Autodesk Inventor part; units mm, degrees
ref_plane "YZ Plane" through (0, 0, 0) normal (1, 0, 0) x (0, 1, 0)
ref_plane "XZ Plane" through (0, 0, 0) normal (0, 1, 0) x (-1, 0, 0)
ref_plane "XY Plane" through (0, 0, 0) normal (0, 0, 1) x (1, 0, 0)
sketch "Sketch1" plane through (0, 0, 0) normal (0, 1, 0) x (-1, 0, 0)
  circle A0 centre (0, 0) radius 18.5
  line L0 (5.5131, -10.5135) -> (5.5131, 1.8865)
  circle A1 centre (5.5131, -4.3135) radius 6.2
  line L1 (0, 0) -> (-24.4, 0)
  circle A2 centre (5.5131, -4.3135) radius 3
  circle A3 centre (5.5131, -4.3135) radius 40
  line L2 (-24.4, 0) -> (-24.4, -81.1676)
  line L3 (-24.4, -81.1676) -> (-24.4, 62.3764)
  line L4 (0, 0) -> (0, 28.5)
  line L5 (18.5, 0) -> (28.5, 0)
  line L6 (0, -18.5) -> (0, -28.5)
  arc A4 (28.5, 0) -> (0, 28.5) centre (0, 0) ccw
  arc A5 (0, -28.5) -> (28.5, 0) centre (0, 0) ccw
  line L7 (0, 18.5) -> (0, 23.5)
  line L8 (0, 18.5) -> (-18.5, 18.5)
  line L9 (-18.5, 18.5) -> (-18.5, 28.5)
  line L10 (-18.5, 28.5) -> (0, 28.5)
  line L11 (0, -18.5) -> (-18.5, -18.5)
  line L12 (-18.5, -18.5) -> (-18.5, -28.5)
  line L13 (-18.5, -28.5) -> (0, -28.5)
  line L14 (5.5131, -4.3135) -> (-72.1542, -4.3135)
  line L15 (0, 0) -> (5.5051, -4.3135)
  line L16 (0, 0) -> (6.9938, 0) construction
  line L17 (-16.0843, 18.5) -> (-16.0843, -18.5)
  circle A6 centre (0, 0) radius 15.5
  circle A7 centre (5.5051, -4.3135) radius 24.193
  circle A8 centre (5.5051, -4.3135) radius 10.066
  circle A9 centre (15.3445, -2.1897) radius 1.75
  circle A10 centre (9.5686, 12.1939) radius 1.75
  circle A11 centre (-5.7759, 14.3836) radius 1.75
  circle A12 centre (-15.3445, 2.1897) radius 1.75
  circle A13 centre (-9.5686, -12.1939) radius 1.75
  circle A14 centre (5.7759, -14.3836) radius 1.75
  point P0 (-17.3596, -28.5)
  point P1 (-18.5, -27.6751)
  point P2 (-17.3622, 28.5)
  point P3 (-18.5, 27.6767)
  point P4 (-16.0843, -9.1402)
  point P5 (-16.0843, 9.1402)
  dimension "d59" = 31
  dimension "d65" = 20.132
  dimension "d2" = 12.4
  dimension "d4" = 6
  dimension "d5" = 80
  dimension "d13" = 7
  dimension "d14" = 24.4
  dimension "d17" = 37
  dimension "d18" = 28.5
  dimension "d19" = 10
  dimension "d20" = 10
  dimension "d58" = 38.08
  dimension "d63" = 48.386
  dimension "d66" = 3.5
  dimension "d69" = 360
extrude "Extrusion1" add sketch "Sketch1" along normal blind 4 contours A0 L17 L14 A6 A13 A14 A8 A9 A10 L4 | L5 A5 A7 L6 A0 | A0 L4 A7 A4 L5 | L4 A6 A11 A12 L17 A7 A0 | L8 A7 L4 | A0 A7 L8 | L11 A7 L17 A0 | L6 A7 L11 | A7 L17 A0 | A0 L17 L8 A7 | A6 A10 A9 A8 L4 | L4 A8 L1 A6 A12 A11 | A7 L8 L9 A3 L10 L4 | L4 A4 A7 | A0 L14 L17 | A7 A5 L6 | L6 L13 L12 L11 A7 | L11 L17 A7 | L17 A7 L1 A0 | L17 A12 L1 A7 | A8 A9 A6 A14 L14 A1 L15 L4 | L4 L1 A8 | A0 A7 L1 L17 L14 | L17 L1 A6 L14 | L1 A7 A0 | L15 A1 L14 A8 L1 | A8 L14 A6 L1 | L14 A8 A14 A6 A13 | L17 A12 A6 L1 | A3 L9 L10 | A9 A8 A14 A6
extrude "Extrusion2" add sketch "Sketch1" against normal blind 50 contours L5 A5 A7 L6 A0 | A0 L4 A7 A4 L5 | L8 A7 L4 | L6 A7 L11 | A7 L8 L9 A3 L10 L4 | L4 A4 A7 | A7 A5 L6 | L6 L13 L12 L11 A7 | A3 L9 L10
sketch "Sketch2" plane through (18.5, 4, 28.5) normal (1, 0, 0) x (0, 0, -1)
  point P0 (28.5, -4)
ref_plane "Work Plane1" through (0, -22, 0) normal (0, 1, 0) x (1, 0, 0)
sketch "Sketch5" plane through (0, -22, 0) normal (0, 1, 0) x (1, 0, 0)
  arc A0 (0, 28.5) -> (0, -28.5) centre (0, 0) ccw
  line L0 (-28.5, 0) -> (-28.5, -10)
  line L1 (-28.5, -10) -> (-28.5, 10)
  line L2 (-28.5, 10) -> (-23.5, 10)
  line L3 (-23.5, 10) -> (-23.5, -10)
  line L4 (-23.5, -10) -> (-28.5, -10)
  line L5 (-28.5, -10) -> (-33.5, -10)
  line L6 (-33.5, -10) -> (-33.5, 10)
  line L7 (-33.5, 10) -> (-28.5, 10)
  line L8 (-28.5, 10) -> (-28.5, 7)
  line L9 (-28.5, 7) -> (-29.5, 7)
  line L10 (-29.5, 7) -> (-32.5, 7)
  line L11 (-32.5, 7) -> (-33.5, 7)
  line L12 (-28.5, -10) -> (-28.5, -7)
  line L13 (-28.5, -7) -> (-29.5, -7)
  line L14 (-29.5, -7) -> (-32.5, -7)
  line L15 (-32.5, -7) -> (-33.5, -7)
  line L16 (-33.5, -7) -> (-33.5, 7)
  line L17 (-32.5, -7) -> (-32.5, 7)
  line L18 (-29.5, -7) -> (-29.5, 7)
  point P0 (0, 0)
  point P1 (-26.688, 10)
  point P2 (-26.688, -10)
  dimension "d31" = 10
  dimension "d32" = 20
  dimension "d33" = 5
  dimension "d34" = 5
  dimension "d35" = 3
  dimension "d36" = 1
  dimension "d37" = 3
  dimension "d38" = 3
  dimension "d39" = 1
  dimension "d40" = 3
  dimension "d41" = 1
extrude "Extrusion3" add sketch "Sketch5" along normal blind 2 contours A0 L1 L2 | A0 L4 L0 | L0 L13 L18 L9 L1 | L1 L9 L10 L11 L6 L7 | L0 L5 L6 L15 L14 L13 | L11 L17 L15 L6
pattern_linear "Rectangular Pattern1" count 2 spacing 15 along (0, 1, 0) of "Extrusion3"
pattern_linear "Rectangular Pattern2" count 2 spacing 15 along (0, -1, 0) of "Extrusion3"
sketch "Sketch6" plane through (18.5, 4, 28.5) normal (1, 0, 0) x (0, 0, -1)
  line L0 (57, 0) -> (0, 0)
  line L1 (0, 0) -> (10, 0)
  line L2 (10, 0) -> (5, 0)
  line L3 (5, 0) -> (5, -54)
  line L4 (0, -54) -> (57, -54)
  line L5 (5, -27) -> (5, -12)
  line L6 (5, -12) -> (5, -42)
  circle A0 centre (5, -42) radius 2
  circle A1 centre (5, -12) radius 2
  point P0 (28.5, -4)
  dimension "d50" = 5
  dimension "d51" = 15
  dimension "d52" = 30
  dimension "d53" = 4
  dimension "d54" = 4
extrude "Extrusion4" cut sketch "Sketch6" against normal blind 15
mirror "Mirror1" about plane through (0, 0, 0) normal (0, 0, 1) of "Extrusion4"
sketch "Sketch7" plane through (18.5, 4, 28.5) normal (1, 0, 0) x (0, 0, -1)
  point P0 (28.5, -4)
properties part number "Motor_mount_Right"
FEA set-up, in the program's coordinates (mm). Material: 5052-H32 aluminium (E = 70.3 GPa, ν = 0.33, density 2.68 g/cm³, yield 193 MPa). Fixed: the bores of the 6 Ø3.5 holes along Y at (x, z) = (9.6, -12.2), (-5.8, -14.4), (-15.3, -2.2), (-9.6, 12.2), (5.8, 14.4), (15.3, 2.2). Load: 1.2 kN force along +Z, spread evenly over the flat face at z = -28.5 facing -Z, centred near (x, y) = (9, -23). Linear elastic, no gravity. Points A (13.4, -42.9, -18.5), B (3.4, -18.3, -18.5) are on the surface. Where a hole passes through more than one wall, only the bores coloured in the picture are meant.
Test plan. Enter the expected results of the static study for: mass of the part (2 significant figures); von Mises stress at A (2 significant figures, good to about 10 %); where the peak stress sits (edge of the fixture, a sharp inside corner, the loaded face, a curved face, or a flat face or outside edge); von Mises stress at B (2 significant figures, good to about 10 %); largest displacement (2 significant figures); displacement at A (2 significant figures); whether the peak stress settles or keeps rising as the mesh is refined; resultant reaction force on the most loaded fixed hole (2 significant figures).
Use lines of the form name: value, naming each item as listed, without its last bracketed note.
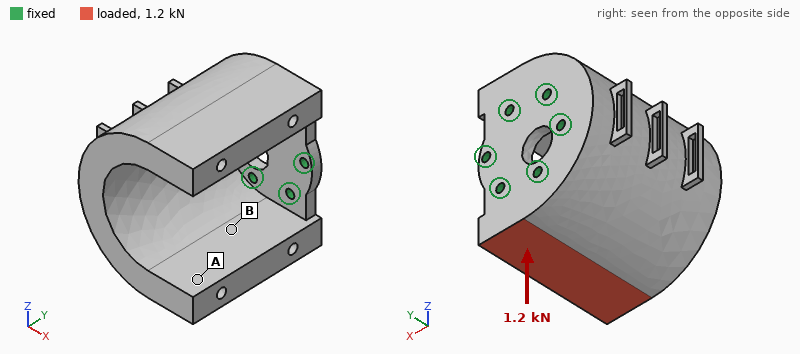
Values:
mass of the part: 170 g
von Mises stress at A: 7.3 MPa
where the peak stress sits: edge of the fixture
von Mises stress at B: 17 MPa
largest displacement: 0.12 mm
displacement at A: 0.096 mm
whether the peak stress settles or keeps rising as the mesh is refined: keeps rising
resultant reaction force on the most loaded fixed hole: 1.1 kN
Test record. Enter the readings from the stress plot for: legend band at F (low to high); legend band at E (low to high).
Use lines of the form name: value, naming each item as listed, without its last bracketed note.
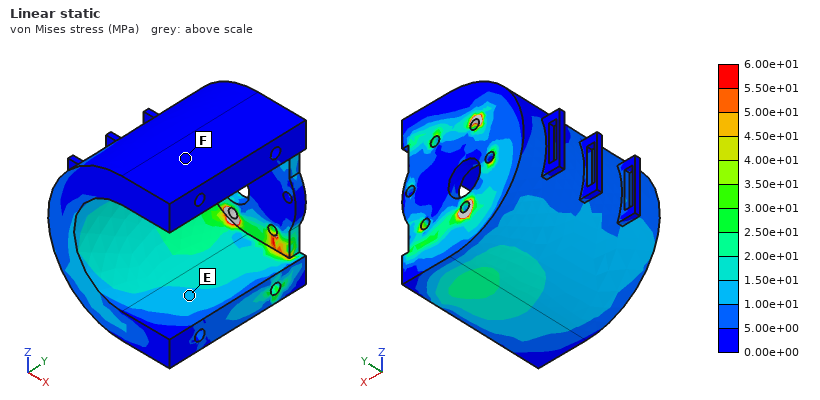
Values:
legend band at F: 0.00e+00 to 5.00e+00 MPa
legend band at E: 1.00e+01 to 1.50e+01 MPa
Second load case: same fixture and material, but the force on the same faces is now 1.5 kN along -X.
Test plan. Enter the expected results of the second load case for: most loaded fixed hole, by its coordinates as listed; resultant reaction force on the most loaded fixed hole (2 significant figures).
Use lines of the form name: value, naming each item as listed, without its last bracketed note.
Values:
most loaded fixed hole, by its coordinates as listed: (9.6, -12.2)
resultant reaction force on the most loaded fixed hole: 1.3 kN
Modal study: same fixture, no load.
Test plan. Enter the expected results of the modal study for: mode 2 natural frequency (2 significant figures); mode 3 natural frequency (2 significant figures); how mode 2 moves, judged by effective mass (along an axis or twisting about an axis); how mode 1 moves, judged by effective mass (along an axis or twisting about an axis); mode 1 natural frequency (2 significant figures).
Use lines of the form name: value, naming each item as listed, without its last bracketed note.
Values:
mode 2 natural frequency: 2800 Hz
mode 3 natural frequency: 5100 Hz
how mode 2 moves, judged by effective mass: along X
how mode 1 moves, judged by effective mass: along Z
mode 1 natural frequency: 2200 Hz
